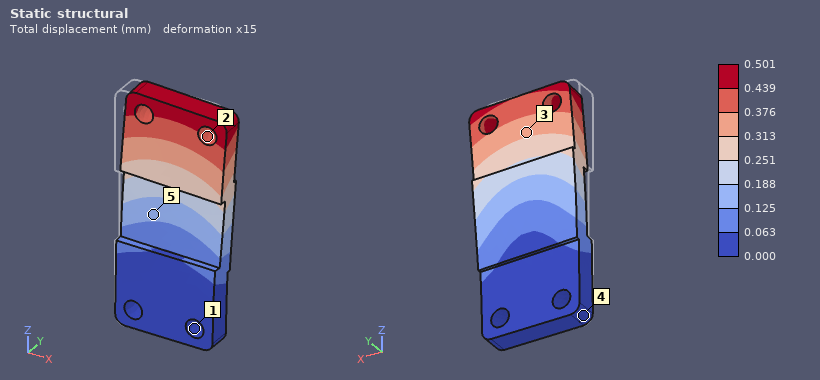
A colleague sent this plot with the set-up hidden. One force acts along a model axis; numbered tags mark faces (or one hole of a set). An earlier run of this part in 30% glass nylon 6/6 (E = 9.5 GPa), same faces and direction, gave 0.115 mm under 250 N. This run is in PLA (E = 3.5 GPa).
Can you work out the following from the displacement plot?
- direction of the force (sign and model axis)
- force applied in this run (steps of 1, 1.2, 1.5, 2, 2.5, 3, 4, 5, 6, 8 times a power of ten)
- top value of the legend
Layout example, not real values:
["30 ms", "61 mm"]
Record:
["+X", "400 N", "0.501 mm"]
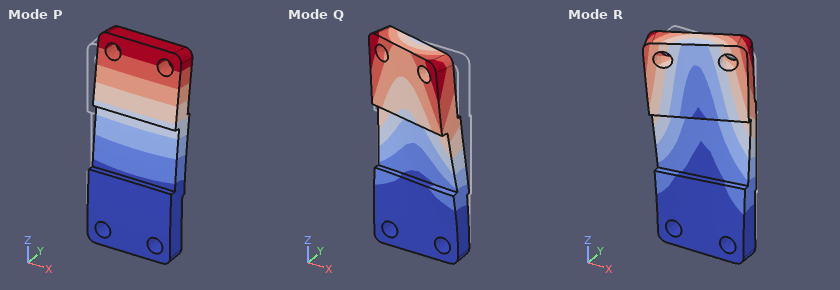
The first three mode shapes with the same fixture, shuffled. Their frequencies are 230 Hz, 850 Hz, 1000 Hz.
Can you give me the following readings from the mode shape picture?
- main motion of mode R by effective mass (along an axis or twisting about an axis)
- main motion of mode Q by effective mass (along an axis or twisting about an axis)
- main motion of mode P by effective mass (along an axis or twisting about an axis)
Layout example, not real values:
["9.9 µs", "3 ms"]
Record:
["along X", "along X", "along Y"]
